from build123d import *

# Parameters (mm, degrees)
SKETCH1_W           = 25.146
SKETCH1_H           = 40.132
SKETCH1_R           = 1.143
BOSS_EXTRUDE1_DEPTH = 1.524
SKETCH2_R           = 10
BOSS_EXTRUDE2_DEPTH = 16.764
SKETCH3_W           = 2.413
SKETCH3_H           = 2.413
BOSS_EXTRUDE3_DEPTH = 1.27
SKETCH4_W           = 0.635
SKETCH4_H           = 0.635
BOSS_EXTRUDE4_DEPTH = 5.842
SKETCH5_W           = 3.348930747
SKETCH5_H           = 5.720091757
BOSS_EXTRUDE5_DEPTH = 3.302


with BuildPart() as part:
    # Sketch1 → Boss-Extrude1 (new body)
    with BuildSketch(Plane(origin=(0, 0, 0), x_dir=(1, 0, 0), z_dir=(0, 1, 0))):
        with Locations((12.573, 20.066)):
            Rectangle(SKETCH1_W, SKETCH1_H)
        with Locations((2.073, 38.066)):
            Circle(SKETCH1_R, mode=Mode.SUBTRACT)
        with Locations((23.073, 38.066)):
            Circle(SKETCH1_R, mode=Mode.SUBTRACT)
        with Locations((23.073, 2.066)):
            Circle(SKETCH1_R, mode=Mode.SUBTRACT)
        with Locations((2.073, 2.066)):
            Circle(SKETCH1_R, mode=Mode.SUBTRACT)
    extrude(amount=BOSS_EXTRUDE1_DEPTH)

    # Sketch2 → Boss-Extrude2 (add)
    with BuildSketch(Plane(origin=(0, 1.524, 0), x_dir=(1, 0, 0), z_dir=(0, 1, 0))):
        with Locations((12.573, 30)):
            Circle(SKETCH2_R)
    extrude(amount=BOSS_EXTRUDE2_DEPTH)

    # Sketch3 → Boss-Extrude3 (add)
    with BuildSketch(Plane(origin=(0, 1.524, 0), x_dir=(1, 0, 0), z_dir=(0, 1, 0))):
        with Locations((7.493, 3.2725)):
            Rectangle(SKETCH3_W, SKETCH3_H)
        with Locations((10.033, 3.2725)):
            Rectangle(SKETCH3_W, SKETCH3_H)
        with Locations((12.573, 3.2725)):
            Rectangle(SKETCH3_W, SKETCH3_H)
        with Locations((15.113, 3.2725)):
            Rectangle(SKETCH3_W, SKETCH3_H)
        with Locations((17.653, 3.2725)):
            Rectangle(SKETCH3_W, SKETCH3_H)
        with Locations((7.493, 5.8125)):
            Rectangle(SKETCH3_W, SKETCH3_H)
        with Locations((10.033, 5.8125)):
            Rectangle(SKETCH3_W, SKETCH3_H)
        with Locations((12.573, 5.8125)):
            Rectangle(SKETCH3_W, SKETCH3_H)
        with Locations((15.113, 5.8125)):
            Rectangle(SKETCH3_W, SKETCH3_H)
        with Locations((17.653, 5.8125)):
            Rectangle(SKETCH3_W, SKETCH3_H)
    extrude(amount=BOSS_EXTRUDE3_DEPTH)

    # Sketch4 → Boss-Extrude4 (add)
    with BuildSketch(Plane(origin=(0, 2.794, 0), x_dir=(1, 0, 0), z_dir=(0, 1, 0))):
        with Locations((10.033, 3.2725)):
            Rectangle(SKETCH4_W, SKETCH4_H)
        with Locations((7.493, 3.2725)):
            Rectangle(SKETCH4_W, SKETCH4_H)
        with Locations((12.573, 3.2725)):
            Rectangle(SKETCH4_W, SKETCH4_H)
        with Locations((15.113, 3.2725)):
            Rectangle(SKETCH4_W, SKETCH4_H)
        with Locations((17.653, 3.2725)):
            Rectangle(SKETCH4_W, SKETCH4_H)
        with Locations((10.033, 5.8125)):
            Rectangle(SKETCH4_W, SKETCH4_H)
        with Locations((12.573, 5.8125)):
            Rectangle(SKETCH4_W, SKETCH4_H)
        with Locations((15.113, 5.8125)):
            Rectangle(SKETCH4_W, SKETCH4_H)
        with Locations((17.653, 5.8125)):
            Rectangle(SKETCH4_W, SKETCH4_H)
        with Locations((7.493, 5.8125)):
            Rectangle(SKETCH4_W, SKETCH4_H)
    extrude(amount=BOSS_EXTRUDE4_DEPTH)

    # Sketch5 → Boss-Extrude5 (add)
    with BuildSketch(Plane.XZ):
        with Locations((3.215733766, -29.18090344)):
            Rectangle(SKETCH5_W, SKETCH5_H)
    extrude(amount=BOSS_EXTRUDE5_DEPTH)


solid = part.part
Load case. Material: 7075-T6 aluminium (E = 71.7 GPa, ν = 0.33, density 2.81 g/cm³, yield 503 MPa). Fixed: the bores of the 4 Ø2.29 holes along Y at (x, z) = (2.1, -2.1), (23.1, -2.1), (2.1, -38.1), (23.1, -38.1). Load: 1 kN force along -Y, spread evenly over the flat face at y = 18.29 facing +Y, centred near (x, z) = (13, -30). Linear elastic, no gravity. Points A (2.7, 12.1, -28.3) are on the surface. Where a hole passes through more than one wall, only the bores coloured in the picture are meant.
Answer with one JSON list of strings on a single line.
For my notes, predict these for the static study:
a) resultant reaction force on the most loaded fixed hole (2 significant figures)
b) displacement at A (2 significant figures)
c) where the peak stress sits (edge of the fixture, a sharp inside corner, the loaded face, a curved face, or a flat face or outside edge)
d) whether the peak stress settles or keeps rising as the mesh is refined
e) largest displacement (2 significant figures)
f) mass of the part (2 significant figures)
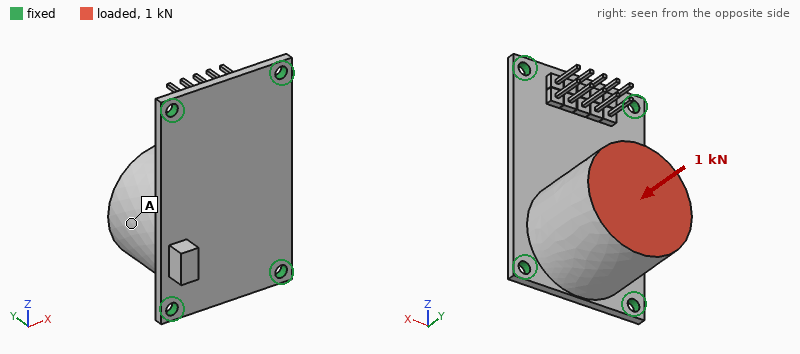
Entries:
["420 N", "0.15 mm", "edge of the fixture", "keeps rising", "0.25 mm", "20 g"]
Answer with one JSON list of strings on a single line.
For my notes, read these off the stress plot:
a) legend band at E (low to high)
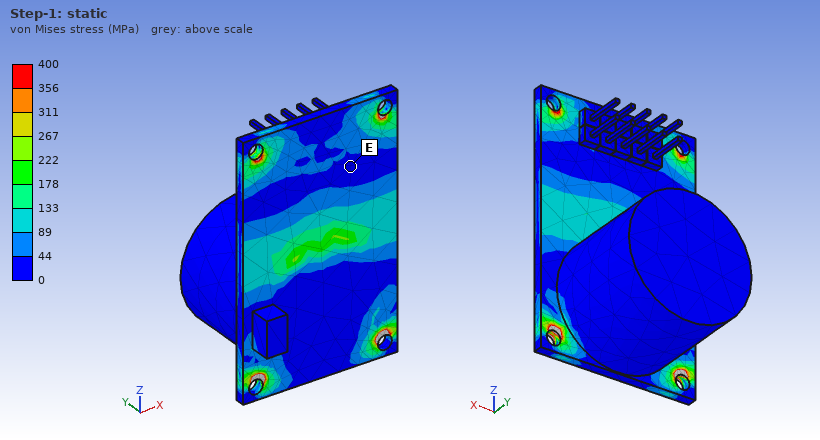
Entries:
["0 to 44 MPa"]
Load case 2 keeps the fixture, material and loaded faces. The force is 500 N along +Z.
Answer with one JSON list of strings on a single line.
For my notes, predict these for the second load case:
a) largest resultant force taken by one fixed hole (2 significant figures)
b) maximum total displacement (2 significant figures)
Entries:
["230 N", "0.33 mm"]
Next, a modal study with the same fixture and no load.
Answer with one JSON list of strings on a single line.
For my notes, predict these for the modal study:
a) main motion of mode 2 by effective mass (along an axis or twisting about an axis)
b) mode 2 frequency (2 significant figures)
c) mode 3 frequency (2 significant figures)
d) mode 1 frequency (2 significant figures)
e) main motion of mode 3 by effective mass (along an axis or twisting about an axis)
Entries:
["along X", "6800 Hz", "9900 Hz", "2300 Hz", "along Y"]
